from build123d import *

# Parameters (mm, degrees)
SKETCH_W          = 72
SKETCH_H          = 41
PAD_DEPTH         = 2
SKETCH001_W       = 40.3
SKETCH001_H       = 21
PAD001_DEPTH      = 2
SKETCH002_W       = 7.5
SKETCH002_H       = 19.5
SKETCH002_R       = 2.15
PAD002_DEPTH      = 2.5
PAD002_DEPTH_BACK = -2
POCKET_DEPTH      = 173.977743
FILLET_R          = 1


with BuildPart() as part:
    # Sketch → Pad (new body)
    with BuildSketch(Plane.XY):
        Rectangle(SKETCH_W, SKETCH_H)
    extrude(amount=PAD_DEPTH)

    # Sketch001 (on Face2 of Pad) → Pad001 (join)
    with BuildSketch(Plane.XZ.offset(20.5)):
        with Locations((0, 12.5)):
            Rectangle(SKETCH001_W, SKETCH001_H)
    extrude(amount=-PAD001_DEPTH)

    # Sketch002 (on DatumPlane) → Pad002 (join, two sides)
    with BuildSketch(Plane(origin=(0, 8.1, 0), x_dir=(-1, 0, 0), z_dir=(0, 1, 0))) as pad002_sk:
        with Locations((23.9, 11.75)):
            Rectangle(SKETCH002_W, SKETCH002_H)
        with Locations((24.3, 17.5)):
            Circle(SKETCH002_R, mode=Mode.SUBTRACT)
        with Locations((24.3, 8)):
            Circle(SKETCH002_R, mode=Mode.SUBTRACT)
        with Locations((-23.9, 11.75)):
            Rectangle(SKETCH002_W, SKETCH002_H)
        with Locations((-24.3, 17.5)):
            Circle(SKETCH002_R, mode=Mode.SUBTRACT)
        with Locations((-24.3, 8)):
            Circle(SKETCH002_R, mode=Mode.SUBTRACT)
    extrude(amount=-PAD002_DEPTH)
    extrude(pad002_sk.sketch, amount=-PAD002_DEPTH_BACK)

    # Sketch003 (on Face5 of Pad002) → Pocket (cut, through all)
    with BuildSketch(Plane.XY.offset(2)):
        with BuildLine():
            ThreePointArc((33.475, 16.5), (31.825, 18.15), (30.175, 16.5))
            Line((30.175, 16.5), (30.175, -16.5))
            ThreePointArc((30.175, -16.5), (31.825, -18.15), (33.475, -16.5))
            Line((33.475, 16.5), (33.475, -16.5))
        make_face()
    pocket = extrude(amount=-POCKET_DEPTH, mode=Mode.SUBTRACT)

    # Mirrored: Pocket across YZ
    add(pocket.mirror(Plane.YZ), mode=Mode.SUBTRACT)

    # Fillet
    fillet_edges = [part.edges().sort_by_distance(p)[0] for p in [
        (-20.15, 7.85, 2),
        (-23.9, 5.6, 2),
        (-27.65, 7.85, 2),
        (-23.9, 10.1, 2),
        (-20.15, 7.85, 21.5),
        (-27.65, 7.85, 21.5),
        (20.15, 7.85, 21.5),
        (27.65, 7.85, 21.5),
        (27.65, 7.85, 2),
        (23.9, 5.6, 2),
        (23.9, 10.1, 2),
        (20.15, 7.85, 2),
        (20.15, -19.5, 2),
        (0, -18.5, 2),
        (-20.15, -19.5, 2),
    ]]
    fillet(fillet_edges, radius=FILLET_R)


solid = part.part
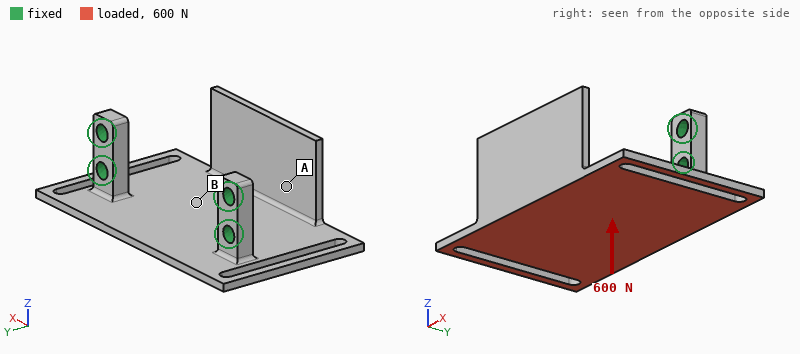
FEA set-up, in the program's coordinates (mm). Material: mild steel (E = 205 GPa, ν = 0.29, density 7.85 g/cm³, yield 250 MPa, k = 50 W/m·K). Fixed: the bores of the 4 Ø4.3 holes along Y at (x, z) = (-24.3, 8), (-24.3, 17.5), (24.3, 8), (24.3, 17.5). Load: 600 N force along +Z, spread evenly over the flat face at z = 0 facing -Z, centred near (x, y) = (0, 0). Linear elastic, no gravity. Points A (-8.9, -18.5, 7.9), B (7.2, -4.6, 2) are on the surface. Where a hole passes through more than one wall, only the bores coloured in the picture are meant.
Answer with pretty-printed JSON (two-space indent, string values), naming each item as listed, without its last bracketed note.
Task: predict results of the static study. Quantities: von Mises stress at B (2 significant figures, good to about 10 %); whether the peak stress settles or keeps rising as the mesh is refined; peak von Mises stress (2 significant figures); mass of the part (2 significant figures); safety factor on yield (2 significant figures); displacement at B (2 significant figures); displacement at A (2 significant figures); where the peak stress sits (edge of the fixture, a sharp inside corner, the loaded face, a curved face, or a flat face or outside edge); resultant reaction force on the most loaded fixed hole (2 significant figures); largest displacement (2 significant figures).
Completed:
{
  "von Mises stress at B": "42 MPa",
  "whether the peak stress settles or keeps rising as the mesh is refined": "settles",
  "peak von Mises stress": "570 MPa",
  "mass of the part": "64 g",
  "safety factor on yield": "0.44",
  "displacement at B": "0.075 mm",
  "displacement at A": "0.18 mm",
  "where the peak stress sits": "a curved face",
  "resultant reaction force on the most loaded fixed hole": "320 N",
  "largest displacement": "0.25 mm"
}
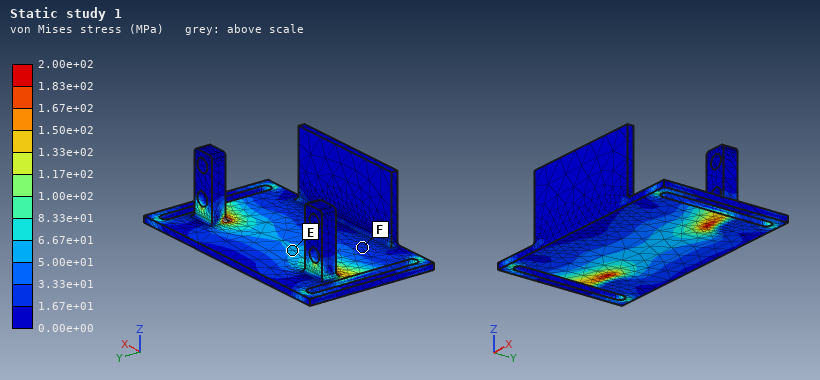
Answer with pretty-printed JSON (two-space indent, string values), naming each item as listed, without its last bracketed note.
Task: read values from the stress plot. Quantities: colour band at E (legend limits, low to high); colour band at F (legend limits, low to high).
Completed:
{
  "colour band at E": "5.00e+01 to 6.67e+01 MPa",
  "colour band at F": "1.67e+01 to 3.33e+01 MPa"
}
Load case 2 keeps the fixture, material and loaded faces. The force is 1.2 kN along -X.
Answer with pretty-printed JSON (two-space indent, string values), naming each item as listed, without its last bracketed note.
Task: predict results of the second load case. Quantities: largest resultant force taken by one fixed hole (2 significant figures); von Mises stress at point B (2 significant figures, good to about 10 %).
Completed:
{
  "largest resultant force taken by one fixed hole": "670 N",
  "von Mises stress at point B": "6.2 MPa"
}
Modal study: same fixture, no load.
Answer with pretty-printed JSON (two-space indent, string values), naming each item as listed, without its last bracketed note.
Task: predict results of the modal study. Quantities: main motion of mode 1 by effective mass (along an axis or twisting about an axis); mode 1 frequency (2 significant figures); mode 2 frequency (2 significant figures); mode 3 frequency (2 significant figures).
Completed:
{
  "main motion of mode 1 by effective mass": "along Z",
  "mode 1 frequency": "940 Hz",
  "mode 2 frequency": "1900 Hz",
  "mode 3 frequency": "2600 Hz"
}
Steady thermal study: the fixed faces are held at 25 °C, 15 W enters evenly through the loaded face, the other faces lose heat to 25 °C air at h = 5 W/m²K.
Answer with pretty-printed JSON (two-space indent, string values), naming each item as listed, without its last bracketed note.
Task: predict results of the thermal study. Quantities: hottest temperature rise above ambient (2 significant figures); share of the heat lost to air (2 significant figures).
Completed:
{
  "hottest temperature rise above ambient": "57 K",
  "share of the heat lost to air": "7.9 %"
}
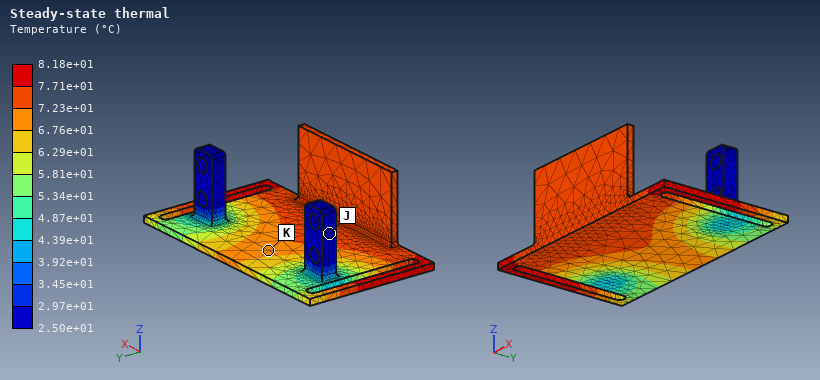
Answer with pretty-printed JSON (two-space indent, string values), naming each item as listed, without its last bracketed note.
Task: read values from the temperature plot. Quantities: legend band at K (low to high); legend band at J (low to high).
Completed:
{
  "legend band at K": "6.76e+01 to 7.23e+01 °C",
  "legend band at J": "2.50e+01 to 2.97e+01 °C"
}
